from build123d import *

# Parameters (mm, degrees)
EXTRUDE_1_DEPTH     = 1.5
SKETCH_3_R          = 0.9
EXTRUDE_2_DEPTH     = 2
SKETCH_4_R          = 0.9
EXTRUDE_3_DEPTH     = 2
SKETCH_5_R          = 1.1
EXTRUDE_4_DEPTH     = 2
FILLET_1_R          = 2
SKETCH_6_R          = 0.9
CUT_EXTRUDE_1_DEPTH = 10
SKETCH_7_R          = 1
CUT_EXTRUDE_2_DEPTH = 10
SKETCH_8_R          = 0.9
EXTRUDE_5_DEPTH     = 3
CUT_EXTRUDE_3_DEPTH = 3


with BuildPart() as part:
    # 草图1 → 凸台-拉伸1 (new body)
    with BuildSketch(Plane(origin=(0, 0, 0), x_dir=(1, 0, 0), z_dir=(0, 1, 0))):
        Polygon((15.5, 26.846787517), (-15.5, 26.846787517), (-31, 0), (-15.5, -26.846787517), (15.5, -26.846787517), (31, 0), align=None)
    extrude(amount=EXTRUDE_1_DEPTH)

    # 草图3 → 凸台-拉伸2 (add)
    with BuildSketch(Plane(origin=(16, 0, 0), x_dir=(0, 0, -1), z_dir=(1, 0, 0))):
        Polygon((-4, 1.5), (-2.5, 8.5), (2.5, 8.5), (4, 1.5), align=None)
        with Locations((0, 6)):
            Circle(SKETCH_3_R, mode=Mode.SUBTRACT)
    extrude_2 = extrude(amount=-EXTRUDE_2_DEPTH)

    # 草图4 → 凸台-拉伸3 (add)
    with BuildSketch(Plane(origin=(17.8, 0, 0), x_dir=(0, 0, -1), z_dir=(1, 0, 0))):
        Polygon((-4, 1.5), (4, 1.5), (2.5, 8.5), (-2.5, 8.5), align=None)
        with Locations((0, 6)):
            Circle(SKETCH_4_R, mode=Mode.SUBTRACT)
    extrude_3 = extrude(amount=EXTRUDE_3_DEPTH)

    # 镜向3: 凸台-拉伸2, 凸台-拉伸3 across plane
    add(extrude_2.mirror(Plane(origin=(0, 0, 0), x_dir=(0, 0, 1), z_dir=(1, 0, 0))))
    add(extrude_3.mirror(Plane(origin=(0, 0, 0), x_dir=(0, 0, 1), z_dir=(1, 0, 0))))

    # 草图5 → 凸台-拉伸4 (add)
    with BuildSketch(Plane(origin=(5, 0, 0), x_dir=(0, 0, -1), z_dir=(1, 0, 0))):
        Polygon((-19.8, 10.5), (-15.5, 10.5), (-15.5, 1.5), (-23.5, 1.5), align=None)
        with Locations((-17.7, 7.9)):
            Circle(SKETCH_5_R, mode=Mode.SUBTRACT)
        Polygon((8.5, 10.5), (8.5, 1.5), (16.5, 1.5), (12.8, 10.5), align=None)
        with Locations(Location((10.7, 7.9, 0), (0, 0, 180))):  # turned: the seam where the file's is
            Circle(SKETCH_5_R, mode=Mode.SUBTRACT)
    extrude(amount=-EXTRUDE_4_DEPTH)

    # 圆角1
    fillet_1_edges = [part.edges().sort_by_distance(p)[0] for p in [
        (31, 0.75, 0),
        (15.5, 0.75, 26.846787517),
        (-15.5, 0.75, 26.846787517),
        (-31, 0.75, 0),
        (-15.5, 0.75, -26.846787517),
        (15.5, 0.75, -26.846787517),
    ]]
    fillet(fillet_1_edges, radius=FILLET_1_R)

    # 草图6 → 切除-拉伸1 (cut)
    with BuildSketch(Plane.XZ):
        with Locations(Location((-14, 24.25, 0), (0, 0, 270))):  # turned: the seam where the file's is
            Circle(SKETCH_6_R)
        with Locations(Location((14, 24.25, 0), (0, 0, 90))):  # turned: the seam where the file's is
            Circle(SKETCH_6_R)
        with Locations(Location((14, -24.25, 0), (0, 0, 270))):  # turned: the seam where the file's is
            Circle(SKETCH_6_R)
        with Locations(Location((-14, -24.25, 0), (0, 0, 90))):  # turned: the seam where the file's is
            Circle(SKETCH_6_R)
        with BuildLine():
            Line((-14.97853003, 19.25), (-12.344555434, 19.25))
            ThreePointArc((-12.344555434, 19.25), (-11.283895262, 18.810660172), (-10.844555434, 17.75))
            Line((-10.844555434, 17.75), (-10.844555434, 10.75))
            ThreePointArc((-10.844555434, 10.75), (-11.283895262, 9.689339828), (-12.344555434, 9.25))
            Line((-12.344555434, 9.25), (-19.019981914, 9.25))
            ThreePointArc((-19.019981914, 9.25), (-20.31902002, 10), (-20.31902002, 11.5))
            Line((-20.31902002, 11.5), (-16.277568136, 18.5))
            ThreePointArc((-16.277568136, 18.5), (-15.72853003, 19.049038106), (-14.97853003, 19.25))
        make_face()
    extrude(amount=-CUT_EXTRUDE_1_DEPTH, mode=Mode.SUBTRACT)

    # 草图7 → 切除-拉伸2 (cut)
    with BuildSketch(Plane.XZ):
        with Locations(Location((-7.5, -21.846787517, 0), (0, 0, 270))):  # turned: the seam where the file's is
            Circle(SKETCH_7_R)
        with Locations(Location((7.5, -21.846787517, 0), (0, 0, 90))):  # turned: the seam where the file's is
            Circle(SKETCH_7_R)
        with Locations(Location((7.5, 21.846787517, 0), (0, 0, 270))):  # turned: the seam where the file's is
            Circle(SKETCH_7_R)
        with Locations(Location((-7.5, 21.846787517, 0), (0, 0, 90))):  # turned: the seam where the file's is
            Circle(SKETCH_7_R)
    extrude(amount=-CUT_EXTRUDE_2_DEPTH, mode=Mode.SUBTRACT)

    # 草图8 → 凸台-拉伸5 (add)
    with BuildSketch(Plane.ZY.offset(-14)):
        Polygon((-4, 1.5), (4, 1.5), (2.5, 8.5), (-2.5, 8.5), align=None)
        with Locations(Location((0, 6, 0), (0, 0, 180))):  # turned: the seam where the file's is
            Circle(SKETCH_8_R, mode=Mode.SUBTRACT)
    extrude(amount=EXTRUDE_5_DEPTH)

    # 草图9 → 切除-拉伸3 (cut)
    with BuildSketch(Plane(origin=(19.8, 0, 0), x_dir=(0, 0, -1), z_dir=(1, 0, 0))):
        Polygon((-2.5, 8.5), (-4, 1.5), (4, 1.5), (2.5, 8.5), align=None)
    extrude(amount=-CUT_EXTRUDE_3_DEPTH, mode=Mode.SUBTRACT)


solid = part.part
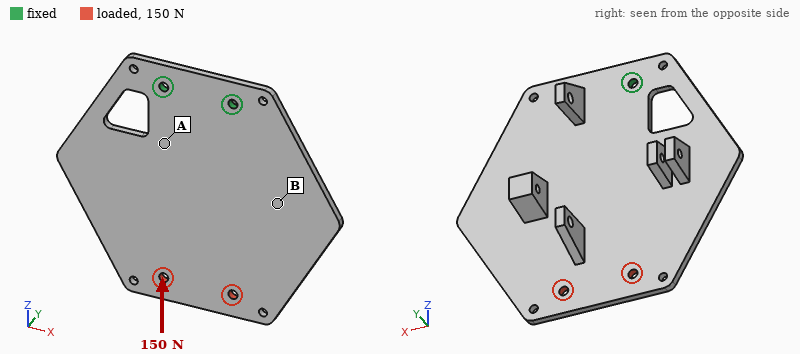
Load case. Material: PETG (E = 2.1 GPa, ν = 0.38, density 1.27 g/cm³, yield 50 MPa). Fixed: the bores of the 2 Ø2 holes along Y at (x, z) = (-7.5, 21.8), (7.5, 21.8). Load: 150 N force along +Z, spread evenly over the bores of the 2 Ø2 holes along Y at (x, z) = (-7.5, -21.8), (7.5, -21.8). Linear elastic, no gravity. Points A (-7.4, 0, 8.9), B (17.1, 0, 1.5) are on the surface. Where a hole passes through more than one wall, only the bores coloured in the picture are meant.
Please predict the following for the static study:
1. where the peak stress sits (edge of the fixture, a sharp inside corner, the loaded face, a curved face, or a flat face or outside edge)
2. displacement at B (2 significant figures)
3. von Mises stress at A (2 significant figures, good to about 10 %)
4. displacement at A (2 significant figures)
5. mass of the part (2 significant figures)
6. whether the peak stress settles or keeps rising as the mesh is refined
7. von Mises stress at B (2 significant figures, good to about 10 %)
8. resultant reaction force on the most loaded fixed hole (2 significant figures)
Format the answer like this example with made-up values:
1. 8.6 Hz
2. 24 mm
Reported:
1. edge of the fixture
2. 0.036 mm
3. 3.9 MPa
4. 0.034 mm
5. 5.3 g
6. keeps rising
7. 1.6 MPa
8. 75 N
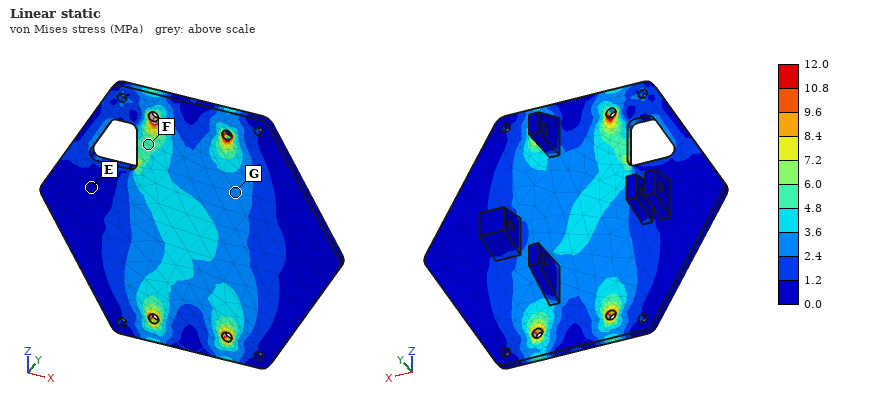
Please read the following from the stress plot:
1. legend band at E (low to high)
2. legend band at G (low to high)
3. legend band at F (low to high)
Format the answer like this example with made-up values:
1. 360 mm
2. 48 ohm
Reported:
1. 0.0 to 1.2 MPa
2. 2.4 to 3.6 MPa
3. 4.8 to 6.0 MPa
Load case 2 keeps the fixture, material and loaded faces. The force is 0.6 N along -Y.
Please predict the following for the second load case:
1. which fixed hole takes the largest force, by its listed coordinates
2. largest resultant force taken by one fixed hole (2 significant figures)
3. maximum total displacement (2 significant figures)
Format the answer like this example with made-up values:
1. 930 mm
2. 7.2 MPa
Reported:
1. (7.5, 21.8)
2. 0.50 N
3. 0.76 mm
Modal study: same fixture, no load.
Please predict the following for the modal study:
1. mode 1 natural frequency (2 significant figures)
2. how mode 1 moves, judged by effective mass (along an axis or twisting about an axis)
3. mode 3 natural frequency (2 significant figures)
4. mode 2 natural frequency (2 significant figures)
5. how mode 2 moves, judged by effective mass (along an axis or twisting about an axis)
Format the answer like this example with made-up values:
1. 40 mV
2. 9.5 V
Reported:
1. 130 Hz
2. along Y
3. 590 Hz
4. 260 Hz
5. twisting about Z
